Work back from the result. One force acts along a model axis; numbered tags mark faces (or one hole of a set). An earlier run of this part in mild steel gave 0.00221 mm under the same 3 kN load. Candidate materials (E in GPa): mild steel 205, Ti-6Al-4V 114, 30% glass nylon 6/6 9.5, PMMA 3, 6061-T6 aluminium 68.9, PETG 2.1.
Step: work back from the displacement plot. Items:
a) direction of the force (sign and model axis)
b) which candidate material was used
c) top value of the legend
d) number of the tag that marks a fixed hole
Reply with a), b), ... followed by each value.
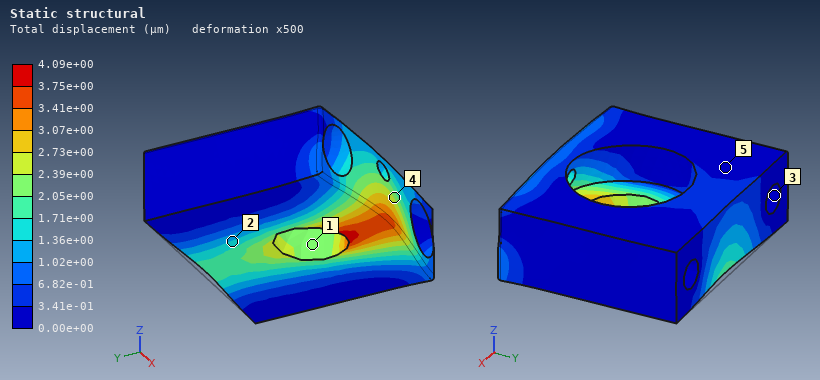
a) -Y
b) Ti-6Al-4V
c) 4.09e+00 µm
d) 3
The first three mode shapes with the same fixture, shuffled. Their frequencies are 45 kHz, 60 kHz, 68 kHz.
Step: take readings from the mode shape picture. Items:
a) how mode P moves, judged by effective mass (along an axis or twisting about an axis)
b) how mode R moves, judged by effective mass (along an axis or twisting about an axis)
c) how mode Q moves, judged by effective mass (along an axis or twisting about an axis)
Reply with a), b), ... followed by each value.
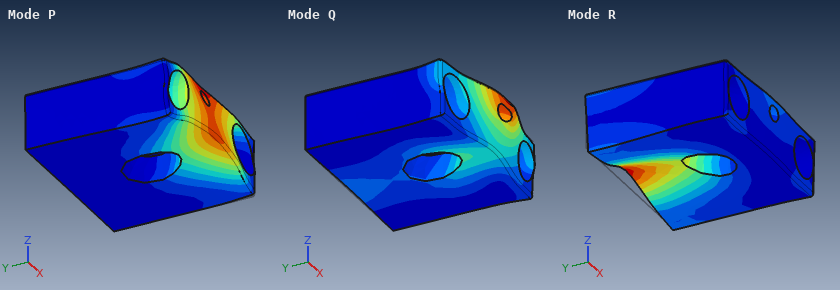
a) along Z
b) along Z
c) along Y
